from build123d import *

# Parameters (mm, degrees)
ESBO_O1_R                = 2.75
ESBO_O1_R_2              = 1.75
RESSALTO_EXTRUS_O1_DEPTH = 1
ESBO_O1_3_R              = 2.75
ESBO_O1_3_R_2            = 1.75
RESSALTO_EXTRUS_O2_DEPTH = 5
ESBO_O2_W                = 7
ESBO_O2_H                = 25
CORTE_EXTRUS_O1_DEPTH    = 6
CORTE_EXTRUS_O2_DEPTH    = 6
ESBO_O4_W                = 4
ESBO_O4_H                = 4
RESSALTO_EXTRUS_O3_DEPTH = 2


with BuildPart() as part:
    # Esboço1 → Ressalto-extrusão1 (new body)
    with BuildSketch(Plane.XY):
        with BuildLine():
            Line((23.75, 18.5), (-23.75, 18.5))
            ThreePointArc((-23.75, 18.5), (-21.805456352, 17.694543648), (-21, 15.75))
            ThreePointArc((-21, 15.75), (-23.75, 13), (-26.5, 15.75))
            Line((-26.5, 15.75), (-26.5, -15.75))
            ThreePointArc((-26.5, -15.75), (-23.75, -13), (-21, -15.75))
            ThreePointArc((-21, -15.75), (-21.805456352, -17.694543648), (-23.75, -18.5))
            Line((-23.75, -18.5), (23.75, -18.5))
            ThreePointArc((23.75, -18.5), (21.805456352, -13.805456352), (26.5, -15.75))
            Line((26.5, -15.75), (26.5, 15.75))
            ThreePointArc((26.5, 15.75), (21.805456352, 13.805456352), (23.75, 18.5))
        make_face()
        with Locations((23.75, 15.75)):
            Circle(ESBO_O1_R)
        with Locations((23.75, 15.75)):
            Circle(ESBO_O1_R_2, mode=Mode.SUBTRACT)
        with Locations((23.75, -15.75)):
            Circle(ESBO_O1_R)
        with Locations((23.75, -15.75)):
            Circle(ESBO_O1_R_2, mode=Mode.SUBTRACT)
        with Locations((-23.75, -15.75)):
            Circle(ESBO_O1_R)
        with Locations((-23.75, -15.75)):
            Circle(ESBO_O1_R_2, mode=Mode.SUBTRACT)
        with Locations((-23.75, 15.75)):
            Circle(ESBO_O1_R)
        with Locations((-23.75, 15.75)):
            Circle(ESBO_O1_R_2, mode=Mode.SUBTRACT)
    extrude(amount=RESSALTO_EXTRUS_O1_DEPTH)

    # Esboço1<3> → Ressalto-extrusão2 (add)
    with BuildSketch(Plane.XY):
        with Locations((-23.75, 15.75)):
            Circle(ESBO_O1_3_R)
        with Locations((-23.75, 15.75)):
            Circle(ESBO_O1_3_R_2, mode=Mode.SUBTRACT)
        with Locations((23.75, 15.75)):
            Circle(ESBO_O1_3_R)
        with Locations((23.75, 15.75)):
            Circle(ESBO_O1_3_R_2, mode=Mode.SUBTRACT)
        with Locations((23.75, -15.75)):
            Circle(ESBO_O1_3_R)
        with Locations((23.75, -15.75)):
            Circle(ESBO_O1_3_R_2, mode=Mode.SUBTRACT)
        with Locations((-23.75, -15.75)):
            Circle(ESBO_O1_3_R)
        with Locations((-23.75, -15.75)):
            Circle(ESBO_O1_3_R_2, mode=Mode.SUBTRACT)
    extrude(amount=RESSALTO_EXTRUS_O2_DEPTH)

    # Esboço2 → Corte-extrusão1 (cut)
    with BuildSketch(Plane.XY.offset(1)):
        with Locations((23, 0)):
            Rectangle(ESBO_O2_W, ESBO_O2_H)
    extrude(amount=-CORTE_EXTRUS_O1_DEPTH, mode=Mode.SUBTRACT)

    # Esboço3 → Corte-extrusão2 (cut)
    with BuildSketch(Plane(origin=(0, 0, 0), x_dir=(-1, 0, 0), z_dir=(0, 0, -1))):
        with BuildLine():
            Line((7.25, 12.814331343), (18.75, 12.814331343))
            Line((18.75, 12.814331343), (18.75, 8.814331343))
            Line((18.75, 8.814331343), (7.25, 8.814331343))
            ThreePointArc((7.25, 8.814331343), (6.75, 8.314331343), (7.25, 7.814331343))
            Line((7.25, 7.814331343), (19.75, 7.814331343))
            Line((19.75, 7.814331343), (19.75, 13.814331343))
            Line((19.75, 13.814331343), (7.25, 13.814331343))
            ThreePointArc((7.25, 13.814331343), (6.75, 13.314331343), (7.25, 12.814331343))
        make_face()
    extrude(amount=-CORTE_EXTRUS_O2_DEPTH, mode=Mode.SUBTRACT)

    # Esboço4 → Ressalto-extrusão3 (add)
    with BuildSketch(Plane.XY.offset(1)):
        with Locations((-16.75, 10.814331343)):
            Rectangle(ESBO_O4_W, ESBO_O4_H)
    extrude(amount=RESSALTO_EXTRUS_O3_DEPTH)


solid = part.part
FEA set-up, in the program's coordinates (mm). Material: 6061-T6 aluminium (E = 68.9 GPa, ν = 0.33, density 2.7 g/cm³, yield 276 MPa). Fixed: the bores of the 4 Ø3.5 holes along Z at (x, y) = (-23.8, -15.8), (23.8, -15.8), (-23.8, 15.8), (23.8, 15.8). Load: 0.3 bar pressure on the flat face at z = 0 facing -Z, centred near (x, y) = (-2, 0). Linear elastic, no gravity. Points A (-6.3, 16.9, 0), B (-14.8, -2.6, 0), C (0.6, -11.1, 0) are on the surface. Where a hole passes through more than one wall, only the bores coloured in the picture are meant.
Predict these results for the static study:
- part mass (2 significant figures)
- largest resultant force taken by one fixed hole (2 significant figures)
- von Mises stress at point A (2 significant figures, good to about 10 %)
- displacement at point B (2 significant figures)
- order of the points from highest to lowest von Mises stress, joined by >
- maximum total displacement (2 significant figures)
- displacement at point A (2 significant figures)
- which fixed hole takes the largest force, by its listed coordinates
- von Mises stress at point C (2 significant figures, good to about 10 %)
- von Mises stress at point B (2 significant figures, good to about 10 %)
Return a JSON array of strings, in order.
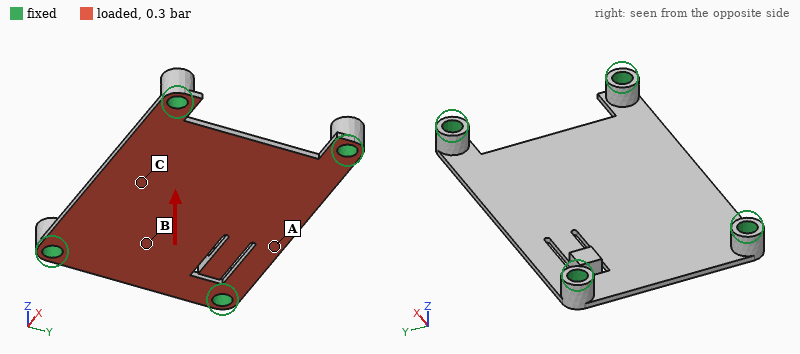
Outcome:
["5.3 g", "16 N", "26 MPa", "47 µm", "A > C > B", "90 µm", "74 µm", "(-23.8, -15.8)", "18 MPa", "7.7 MPa"]
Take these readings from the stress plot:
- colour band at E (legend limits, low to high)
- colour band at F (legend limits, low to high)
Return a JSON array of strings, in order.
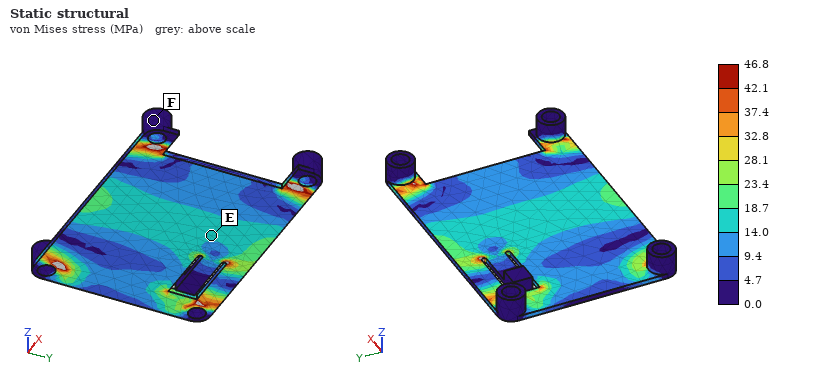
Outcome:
["14.0 to 18.7 MPa", "0.0 to 4.7 MPa"]
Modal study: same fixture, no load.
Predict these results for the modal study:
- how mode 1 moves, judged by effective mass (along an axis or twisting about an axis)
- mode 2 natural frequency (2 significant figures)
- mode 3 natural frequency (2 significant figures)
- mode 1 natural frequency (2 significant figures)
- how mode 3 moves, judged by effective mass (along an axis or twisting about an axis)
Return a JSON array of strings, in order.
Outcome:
["along Z", "2500 Hz", "3300 Hz", "1900 Hz", "twisting about X"]
